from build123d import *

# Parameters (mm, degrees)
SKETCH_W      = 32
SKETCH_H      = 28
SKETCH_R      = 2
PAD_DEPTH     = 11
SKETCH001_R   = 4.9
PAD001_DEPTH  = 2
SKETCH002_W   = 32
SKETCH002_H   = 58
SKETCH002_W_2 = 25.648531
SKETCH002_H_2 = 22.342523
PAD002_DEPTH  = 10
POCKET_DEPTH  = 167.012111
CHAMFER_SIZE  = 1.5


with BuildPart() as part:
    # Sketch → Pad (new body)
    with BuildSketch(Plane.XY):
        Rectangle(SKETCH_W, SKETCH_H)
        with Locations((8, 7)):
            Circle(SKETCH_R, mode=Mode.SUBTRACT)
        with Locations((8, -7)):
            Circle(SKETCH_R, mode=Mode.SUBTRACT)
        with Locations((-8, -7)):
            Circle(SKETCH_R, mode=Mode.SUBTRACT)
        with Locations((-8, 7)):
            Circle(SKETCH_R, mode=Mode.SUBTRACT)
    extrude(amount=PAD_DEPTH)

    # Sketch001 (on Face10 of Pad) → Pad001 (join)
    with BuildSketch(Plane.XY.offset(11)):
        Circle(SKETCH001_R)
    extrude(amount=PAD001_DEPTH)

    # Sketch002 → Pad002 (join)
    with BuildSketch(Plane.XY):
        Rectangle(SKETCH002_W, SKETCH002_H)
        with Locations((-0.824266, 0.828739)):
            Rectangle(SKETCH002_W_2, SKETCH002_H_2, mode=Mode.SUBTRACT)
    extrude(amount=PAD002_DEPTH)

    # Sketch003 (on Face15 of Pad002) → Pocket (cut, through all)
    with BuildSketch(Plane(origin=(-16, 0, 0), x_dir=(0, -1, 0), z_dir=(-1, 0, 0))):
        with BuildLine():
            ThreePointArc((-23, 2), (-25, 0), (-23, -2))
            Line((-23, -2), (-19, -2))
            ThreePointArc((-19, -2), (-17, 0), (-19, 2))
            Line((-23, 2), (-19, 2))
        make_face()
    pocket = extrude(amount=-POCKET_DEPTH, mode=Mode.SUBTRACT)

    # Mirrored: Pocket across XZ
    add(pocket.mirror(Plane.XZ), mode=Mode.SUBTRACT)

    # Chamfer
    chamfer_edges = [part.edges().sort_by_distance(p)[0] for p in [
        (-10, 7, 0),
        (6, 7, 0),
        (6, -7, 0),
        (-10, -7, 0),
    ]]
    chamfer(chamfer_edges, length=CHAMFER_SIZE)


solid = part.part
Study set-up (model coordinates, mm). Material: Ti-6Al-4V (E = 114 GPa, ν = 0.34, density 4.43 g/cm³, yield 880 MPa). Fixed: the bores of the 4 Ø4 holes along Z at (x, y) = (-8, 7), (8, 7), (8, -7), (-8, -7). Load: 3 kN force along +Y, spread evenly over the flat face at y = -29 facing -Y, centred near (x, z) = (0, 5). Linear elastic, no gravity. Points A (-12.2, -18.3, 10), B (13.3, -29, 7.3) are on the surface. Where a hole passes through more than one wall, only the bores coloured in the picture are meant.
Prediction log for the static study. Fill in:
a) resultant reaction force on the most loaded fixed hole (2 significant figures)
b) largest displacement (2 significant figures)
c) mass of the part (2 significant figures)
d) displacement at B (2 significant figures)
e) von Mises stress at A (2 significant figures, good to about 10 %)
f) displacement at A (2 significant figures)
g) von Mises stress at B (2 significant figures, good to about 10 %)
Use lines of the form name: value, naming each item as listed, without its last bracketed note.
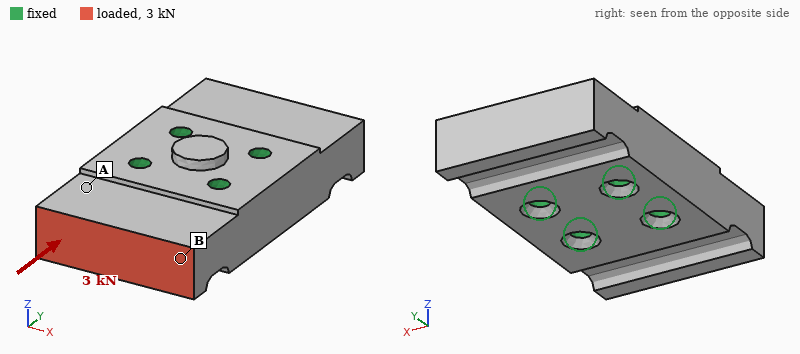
resultant reaction force on the most loaded fixed hole: 1.3 kN
largest displacement: 4.3 µm
mass of the part: 80 g
displacement at B: 2.8 µm
von Mises stress at A: 5.2 MPa
displacement at A: 0.88 µm
von Mises stress at B: 10 MPa
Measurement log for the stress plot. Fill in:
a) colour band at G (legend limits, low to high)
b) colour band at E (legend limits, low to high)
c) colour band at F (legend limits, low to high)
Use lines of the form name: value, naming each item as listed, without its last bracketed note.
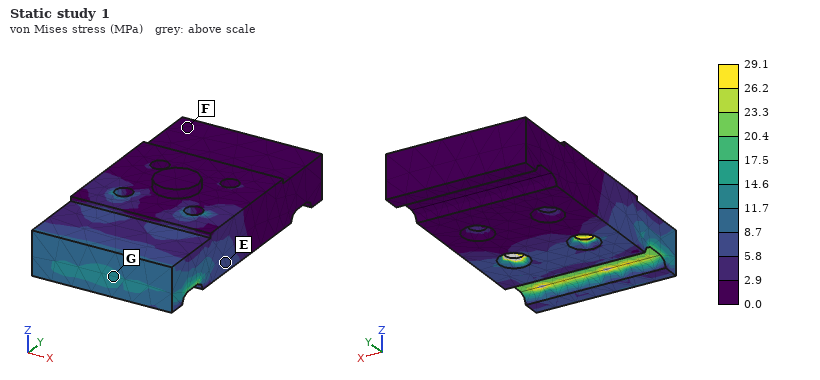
colour band at G: 11.7 to 14.6 MPa
colour band at E: 5.8 to 8.7 MPa
colour band at F: 0.0 to 2.9 MPa
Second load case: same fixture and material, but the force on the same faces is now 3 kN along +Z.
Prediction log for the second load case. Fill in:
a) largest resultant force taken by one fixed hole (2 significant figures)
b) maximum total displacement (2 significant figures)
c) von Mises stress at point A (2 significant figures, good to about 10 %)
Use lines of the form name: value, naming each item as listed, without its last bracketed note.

largest resultant force taken by one fixed hole: 2.1 kN
maximum total displacement: 49 µm
von Mises stress at point A: 79 MPa
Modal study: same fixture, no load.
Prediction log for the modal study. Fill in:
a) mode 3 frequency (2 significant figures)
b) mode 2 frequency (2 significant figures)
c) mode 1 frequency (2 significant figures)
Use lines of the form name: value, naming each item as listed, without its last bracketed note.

mode 3 frequency: 22 kHz
mode 2 frequency: 15 kHz
mode 1 frequency: 15 kHz
